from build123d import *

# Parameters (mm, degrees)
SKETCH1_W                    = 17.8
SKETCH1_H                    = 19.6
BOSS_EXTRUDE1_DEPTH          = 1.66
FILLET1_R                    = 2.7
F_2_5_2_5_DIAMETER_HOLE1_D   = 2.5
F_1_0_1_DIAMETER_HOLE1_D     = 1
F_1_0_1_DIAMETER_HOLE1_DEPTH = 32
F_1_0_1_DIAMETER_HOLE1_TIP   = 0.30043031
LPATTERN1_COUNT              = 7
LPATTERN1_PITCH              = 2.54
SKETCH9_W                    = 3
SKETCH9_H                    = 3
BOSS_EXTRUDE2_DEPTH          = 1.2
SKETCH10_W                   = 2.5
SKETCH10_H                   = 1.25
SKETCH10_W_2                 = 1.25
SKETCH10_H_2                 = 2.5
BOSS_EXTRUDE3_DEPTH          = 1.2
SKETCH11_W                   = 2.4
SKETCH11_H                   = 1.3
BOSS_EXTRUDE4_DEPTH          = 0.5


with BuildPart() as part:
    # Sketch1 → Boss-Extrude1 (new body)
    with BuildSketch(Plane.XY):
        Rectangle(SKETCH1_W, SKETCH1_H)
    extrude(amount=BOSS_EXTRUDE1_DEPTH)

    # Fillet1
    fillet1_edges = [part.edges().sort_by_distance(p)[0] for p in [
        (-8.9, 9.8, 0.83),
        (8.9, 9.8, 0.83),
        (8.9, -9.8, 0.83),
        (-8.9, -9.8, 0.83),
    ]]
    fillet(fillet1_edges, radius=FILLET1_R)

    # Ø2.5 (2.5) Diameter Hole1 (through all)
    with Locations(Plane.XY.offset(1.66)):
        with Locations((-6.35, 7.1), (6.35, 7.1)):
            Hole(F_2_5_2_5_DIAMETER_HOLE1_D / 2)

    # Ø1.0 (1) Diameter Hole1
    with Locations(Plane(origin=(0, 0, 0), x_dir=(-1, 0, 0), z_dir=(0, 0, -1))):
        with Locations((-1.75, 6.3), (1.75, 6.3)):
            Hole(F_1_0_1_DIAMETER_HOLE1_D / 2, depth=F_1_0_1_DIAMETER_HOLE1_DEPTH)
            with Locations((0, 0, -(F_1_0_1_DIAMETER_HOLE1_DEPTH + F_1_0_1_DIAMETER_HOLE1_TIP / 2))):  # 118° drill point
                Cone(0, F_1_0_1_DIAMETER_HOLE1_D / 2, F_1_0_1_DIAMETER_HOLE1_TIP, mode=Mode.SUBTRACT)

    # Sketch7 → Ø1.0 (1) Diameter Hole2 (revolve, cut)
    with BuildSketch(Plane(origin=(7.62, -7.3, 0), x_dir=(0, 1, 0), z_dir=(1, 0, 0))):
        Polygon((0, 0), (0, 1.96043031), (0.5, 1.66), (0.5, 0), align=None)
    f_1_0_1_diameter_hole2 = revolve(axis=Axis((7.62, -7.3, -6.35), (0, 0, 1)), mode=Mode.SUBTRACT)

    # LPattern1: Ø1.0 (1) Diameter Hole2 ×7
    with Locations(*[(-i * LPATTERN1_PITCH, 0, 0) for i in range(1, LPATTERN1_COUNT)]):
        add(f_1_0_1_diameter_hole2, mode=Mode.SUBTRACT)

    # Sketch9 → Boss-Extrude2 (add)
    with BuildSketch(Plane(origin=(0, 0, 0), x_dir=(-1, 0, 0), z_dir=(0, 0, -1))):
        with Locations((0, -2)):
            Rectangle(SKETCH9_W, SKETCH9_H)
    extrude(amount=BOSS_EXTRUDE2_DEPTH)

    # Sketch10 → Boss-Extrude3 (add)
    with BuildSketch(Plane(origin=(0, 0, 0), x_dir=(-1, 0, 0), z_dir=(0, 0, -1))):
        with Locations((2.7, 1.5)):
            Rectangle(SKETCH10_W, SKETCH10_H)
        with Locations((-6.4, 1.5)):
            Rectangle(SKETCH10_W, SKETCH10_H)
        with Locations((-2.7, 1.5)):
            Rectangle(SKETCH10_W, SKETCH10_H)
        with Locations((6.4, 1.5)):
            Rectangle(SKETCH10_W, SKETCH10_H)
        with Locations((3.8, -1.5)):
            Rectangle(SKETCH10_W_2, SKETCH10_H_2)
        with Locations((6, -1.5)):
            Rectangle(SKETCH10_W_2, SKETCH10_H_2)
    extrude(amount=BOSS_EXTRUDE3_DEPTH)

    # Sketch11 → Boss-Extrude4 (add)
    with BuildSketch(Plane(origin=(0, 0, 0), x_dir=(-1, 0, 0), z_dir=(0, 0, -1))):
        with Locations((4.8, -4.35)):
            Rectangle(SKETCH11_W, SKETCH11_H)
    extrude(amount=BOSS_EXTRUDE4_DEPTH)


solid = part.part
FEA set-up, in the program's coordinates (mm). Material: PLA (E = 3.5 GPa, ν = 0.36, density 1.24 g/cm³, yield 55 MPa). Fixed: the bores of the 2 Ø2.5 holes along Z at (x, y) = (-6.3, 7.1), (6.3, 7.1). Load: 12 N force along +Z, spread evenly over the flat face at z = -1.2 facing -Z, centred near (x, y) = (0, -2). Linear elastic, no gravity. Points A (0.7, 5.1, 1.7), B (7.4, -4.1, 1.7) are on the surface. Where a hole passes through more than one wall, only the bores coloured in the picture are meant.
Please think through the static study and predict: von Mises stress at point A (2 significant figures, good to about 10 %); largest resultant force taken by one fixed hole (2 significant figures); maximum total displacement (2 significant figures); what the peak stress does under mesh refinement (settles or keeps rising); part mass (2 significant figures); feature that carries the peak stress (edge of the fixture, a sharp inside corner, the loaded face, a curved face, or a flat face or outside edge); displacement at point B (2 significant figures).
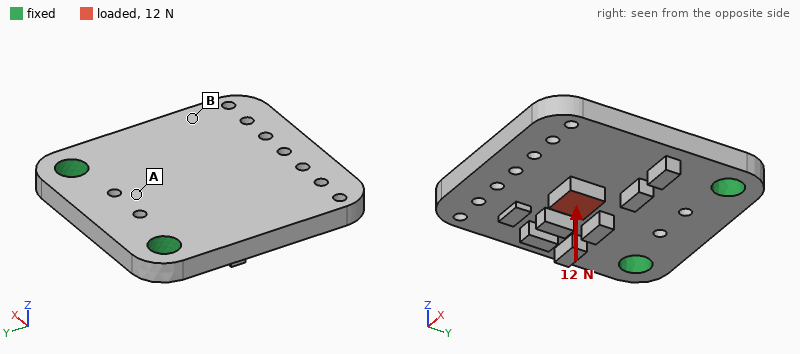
6.3 MPa
6.0 N
0.29 mm
keeps rising
0.71 g
edge of the fixture
0.15 mm
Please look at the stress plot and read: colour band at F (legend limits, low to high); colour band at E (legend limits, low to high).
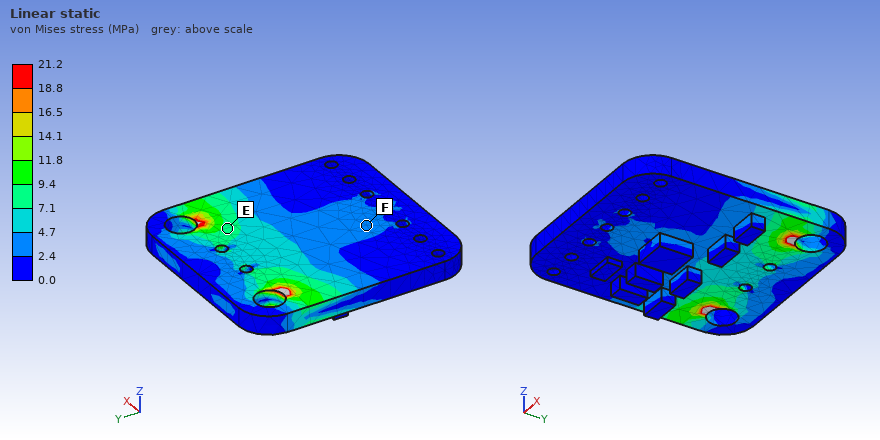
2.4 to 4.7 MPa
7.1 to 9.4 MPa
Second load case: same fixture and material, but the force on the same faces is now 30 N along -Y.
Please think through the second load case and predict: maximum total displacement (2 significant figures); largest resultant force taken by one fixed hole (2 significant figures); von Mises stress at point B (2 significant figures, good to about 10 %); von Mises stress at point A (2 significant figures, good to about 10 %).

0.26 mm
16 N
1.4 MPa
4.1 MPa
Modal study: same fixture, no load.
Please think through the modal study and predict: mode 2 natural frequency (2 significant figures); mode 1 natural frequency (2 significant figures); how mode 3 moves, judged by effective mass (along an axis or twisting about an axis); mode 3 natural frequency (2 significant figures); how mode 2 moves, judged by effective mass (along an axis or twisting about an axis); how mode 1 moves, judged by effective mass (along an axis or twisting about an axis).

4200 Hz
1700 Hz
along Z
9700 Hz
twisting about Y
along Z
